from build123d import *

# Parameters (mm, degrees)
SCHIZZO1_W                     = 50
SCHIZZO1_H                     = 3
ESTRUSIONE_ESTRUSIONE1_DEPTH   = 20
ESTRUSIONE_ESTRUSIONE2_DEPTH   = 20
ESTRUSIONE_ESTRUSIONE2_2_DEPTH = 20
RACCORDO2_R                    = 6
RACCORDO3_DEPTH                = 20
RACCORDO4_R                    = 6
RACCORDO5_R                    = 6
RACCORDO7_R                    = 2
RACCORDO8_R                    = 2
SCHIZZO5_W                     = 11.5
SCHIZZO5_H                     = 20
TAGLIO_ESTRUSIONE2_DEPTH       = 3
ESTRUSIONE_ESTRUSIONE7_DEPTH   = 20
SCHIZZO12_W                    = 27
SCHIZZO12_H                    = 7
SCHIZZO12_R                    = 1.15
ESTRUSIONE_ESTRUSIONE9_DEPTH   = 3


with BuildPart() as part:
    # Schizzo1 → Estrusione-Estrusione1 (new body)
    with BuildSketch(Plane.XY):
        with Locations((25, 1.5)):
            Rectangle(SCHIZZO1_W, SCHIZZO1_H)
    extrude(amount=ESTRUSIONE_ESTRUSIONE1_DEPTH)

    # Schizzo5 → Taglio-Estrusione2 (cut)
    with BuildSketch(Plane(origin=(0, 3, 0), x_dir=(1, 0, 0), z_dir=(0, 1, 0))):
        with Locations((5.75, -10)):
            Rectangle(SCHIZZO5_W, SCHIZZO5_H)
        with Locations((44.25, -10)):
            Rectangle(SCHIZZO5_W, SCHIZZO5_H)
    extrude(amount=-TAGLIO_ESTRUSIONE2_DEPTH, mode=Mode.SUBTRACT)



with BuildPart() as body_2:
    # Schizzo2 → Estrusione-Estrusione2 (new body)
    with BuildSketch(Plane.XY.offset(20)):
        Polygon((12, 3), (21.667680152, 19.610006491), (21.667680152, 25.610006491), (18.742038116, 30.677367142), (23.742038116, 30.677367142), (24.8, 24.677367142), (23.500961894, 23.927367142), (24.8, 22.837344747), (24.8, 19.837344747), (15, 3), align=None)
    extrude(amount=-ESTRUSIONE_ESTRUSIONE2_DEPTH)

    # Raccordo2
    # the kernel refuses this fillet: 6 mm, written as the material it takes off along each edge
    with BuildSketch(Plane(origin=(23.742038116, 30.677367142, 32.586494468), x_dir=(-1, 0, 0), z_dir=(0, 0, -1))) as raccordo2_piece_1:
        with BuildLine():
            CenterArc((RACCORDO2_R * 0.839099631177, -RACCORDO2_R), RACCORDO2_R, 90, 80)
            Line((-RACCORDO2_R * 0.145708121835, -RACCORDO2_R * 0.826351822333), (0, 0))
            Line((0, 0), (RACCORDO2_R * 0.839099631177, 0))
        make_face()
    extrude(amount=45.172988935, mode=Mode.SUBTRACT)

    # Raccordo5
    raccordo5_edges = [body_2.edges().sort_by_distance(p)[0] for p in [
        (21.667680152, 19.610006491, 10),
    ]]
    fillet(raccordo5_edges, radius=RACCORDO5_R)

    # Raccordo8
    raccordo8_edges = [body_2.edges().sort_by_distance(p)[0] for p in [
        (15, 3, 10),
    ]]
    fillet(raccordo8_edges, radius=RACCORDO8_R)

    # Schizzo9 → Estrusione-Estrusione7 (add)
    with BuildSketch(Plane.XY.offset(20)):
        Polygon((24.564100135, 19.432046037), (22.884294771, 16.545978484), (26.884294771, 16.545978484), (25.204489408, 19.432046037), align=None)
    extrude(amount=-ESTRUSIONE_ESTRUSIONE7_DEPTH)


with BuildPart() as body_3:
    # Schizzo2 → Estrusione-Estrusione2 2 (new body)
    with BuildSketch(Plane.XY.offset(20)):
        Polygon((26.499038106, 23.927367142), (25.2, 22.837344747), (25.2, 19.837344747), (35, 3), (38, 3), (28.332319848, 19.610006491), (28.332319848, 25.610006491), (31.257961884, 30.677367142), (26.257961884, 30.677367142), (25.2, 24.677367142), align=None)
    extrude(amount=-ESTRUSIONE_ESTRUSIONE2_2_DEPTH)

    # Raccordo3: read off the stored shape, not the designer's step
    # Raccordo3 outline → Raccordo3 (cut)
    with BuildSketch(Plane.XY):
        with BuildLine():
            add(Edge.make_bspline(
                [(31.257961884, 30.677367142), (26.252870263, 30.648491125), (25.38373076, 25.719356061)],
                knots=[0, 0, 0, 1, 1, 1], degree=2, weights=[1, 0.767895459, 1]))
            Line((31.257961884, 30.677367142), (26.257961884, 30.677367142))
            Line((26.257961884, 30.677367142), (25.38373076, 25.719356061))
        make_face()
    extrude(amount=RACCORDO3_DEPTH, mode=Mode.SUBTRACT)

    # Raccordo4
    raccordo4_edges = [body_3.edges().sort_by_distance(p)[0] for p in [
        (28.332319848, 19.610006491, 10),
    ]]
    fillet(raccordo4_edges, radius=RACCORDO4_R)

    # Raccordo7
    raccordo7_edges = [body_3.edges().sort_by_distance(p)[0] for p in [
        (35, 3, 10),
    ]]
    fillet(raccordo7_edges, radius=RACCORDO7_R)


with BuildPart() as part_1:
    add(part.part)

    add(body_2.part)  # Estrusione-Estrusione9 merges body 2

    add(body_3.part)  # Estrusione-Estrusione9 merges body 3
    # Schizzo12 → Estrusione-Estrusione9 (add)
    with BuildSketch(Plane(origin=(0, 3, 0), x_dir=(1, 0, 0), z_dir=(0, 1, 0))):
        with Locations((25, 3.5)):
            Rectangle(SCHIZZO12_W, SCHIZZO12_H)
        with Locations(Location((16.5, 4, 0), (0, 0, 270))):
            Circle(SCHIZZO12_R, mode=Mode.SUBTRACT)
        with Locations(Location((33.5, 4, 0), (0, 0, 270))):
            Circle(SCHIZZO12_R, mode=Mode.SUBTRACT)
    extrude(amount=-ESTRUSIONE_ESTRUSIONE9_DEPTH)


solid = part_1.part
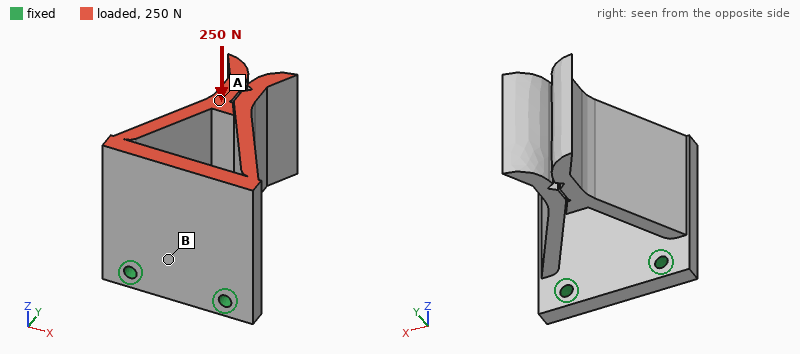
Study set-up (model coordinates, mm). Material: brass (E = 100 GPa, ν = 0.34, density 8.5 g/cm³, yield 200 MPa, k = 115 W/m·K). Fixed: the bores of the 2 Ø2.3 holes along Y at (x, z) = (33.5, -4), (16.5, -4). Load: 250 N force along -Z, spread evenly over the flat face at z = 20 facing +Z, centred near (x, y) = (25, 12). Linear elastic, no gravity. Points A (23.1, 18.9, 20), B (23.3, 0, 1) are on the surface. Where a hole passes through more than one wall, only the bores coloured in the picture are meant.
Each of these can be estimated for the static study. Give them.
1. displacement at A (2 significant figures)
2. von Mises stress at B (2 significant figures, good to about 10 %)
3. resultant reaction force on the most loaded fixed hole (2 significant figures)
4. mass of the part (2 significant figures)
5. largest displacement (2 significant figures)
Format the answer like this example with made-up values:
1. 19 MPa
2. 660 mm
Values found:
1. 0.11 mm
2. 33 MPa
3. 130 N
4. 48 g
5. 0.14 mm
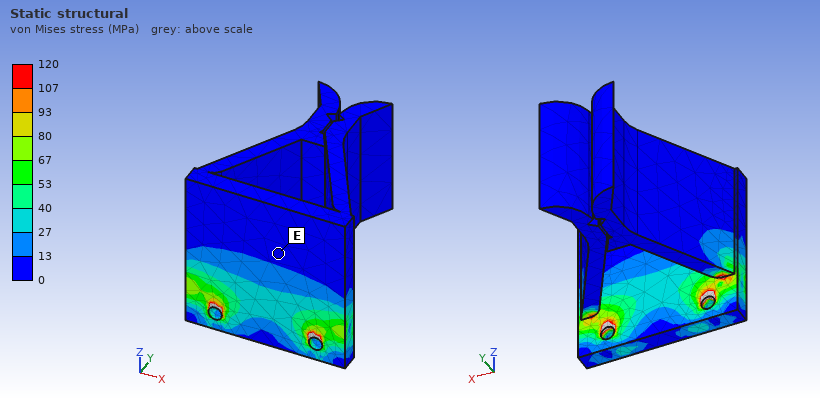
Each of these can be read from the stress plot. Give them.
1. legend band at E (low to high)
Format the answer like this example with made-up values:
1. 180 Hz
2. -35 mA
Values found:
1. 0 to 13 MPa
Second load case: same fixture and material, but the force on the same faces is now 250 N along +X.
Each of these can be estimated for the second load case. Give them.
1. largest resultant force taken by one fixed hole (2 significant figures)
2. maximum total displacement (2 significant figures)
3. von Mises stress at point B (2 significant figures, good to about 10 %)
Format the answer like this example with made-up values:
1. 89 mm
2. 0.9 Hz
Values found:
1. 370 N
2. 0.25 mm
3. 9.1 MPa
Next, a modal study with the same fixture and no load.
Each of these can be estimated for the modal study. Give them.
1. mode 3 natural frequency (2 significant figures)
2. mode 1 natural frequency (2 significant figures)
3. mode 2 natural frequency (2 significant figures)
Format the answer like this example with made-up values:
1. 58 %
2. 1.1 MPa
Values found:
1. 1100 Hz
2. 960 Hz
3. 1000 Hz
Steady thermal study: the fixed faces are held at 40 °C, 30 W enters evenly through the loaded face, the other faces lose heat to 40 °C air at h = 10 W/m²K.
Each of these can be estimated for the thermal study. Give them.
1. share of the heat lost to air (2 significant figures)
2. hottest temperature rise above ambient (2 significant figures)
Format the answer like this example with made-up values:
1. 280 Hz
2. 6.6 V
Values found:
1. 7.1 %
2. 73 K
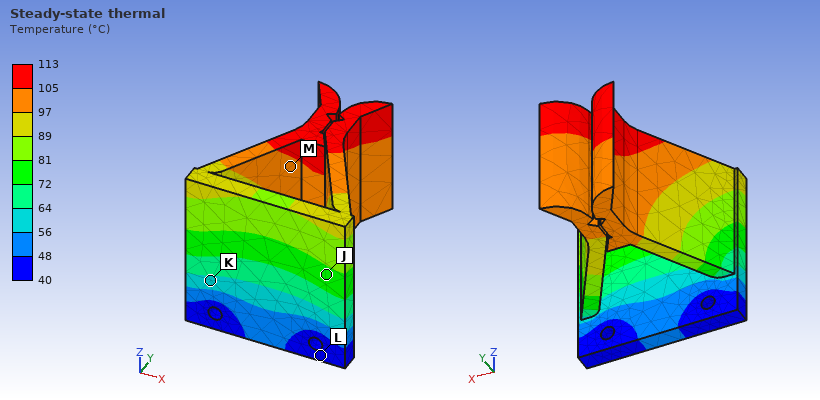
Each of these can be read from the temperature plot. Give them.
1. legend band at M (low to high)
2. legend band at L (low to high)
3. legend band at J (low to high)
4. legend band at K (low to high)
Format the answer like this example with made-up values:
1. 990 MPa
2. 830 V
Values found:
1. 97 to 105 °C
2. 40 to 48 °C
3. 72 to 81 °C
4. 56 to 64 °C
